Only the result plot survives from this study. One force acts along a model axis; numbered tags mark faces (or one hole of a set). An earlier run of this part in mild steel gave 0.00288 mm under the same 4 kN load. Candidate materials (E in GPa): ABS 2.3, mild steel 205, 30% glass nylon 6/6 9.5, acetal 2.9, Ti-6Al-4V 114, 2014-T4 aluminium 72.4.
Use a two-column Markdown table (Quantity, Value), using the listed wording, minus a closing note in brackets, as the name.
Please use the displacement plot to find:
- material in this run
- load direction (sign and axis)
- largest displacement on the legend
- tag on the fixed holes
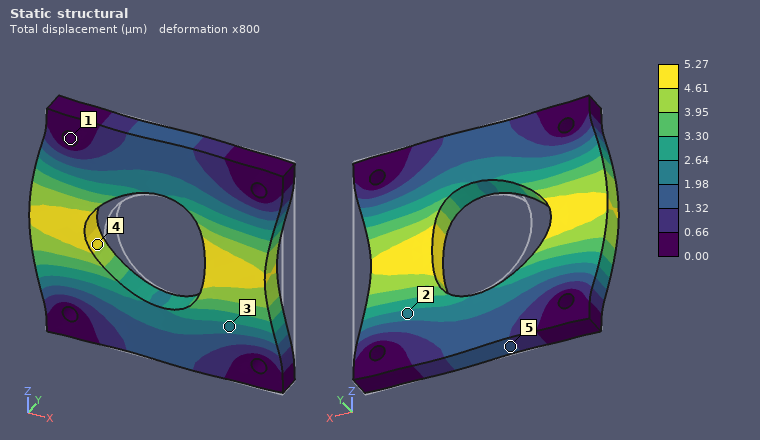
| Quantity | Value |
|---|---|
| material in this run | Ti-6Al-4V |
| load direction | -X |
| largest displacement on the legend | 5.27 µm |
| tag on the fixed holes | 1 |
